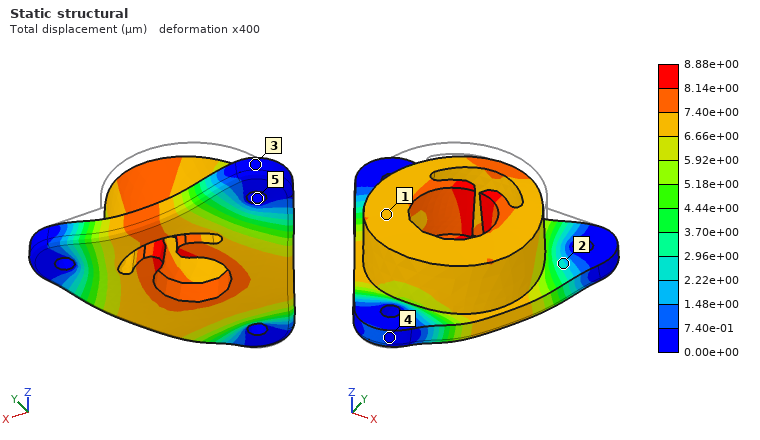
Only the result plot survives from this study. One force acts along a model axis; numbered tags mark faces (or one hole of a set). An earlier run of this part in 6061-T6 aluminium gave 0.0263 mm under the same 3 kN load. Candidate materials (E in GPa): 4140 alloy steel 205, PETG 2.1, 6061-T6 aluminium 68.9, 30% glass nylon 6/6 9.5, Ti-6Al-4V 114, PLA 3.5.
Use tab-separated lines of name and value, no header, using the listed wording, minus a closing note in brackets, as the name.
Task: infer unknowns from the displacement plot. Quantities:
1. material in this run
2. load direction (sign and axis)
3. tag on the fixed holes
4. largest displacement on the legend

material in this run	4140 alloy steel
load direction	-Z
tag on the fixed holes	5
largest displacement on the legend	8.88e+00 µm
